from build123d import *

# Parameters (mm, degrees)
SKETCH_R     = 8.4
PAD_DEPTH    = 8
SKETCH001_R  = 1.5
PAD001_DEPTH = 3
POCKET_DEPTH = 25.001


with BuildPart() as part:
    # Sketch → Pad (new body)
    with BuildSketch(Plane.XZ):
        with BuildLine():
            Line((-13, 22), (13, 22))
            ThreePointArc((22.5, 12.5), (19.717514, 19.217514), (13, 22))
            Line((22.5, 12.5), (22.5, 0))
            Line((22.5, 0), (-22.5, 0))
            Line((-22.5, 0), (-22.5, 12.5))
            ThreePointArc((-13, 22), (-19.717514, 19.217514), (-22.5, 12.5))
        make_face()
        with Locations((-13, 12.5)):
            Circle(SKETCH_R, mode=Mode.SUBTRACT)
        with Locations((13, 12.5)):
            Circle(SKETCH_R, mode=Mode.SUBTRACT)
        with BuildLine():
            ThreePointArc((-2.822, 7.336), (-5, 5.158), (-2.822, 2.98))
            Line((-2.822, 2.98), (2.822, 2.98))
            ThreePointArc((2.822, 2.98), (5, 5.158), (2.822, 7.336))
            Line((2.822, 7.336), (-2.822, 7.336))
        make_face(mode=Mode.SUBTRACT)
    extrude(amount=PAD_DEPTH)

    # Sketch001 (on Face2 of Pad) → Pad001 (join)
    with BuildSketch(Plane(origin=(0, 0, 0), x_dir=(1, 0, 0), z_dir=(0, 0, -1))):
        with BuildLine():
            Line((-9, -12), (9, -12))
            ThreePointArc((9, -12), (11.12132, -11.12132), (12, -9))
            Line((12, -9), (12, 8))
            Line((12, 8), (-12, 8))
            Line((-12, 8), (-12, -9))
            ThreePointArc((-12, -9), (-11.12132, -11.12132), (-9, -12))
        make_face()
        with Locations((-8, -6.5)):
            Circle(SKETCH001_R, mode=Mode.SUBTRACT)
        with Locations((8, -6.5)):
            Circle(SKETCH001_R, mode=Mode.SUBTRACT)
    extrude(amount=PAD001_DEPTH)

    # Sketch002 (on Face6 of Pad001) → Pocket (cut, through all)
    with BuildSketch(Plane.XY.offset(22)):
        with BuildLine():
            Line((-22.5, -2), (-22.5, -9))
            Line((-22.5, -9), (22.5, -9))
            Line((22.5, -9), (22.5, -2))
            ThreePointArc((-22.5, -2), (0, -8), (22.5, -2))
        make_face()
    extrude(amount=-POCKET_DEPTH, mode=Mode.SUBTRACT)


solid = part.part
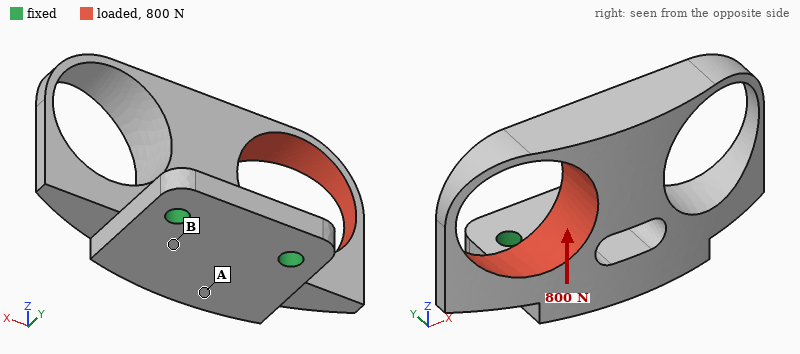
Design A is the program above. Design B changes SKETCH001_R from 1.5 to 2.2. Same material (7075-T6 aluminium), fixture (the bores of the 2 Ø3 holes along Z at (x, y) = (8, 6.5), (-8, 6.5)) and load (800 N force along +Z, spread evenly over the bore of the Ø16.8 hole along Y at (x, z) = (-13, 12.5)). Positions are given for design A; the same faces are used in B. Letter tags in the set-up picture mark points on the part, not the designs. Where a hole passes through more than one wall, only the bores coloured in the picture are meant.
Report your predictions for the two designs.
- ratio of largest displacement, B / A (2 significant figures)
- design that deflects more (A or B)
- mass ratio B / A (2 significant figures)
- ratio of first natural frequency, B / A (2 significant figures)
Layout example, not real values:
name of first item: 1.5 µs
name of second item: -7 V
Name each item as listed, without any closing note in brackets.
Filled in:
ratio of largest displacement, B / A: 0.83
design that deflects more: A
mass ratio B / A: 0.99
ratio of first natural frequency, B / A: 1.1
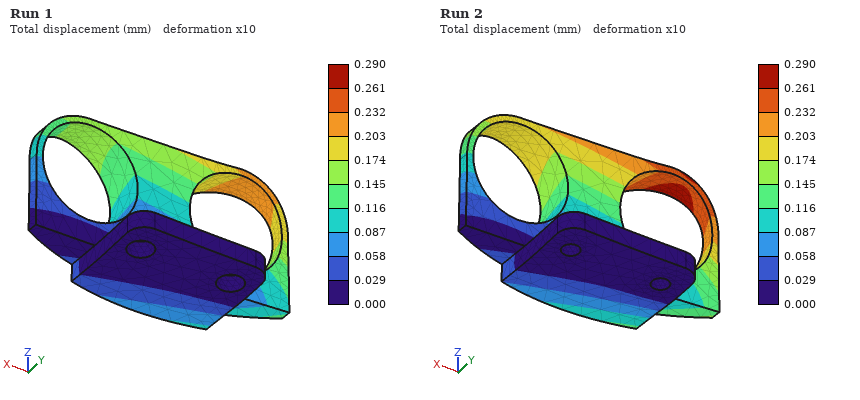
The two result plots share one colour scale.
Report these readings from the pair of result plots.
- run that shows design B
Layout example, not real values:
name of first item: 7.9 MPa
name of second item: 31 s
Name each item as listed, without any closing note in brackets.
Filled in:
run that shows design B: Run 1
